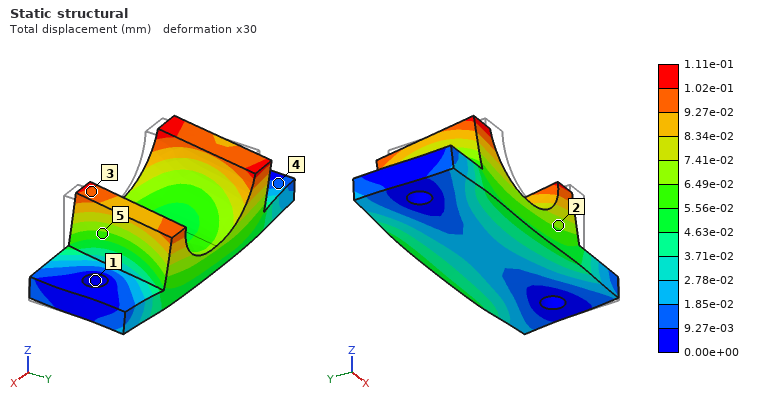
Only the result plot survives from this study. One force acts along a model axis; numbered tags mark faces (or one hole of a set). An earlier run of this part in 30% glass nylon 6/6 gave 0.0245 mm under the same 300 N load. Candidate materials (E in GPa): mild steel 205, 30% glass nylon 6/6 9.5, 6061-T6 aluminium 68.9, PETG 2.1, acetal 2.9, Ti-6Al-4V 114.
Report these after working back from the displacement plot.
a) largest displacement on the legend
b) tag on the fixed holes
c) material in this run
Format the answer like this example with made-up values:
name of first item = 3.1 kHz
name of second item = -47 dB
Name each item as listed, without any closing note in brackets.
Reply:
largest displacement on the legend = 1.11e-01 mm
tag on the fixed holes = 1
material in this run = PETG
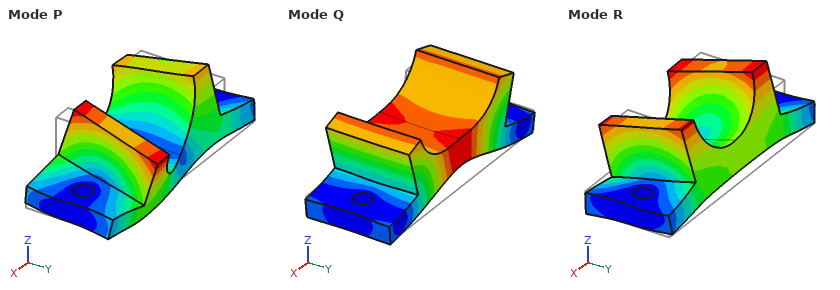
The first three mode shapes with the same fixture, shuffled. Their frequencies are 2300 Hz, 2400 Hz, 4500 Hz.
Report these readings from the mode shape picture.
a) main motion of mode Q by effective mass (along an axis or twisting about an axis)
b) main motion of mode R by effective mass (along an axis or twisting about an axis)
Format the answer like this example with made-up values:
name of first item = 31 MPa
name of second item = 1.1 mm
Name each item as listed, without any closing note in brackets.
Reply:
main motion of mode Q by effective mass = along Z
main motion of mode R by effective mass = along Y
